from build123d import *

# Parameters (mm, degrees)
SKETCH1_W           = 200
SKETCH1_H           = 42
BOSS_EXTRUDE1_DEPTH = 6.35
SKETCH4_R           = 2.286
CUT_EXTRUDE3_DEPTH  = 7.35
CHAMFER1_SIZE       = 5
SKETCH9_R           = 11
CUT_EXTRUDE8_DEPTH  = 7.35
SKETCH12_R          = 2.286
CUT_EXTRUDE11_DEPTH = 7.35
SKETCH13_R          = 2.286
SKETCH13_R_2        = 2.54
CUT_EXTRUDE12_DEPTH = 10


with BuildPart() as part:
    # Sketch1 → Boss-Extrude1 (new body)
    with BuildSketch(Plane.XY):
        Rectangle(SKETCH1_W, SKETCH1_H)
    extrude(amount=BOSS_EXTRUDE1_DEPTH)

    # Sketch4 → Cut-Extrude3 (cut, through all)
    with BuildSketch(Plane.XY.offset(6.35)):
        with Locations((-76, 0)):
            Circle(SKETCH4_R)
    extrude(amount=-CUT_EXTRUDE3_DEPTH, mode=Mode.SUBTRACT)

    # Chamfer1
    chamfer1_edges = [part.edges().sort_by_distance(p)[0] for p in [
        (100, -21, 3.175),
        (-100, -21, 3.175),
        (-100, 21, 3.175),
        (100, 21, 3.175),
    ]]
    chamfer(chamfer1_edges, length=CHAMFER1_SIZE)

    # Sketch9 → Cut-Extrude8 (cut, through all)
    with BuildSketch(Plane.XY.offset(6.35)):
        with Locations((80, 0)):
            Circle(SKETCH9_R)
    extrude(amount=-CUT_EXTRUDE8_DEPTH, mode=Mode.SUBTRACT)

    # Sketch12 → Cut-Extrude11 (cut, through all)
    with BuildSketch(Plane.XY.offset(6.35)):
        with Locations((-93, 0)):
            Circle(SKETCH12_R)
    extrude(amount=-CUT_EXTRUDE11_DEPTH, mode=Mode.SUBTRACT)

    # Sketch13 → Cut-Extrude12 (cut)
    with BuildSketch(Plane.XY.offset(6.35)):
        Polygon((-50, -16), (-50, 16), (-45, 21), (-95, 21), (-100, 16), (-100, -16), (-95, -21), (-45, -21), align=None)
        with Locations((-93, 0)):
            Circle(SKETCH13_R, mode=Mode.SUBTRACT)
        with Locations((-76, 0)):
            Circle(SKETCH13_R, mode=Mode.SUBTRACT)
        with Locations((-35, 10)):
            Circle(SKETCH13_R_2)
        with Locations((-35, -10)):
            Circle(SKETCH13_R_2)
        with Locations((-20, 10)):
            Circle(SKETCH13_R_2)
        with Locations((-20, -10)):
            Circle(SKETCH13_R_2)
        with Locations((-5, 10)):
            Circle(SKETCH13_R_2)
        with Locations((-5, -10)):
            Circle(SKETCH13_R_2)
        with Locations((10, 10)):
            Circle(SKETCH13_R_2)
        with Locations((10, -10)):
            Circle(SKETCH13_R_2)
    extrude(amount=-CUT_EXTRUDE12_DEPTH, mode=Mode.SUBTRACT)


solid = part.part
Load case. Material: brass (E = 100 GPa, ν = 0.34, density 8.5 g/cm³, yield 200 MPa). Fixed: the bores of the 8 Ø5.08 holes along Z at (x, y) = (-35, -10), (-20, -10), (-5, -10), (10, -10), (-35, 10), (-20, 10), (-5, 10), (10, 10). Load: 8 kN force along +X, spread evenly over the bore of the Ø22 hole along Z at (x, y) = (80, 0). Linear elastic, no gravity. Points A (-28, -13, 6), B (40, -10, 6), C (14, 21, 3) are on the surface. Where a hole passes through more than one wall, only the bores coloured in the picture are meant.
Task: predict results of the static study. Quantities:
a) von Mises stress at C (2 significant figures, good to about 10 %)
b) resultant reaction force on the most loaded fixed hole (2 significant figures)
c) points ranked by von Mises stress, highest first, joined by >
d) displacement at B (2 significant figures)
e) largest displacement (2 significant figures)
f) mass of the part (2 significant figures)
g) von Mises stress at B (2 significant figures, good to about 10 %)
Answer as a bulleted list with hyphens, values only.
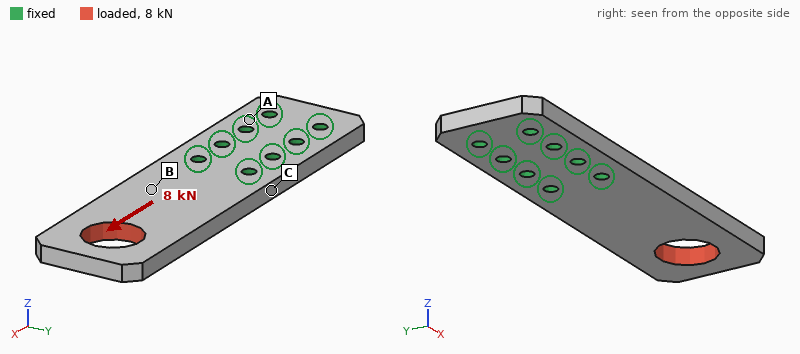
- 18 MPa
- 3.3 kN
- B > C > A
- 9.7 µm
- 38 µm
- 310 g
- 30 MPa
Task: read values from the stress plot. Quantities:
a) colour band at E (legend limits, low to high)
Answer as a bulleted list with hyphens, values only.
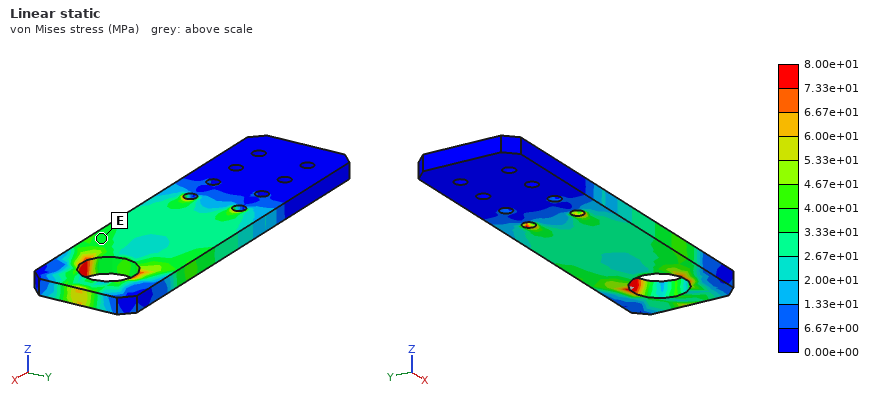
- 3.33e+01 to 4.00e+01 MPa
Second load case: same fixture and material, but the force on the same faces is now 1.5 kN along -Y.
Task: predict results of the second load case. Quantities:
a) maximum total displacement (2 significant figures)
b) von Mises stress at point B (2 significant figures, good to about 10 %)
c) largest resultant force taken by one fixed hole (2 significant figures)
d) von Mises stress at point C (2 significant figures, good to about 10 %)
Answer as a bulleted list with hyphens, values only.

- 98 µm
- 19 MPa
- 3.3 kN
- 41 MPa
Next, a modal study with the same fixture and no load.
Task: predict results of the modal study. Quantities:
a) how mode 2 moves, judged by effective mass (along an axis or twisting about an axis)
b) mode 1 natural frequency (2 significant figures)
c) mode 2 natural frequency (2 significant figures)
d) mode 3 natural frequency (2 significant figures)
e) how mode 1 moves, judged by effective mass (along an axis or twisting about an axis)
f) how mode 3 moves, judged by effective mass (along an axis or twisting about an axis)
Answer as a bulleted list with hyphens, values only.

- twisting about X
- 500 Hz
- 1900 Hz
- 2500 Hz
- along Z
- along Y
